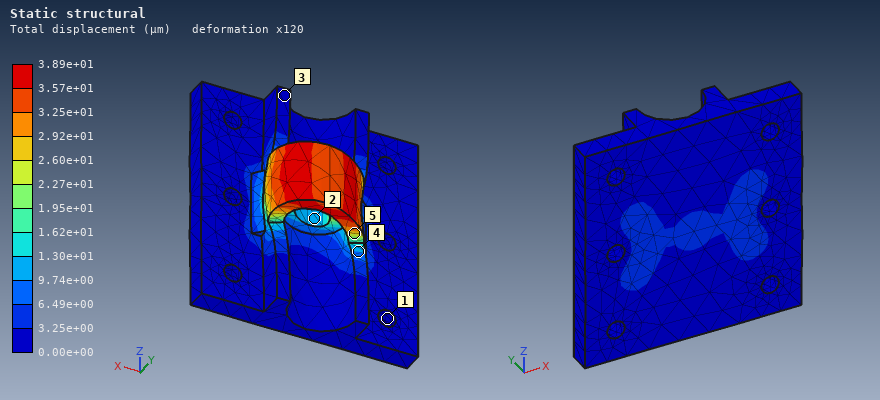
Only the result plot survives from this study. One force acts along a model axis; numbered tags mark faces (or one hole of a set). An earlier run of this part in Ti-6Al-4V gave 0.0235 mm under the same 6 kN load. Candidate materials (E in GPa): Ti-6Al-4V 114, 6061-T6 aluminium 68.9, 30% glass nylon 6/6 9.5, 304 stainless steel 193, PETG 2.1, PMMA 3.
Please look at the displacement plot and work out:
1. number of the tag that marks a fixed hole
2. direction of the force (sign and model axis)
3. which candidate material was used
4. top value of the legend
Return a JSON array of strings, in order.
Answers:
["1", "+X", "6061-T6 aluminium", "3.89e+01 µm"]
